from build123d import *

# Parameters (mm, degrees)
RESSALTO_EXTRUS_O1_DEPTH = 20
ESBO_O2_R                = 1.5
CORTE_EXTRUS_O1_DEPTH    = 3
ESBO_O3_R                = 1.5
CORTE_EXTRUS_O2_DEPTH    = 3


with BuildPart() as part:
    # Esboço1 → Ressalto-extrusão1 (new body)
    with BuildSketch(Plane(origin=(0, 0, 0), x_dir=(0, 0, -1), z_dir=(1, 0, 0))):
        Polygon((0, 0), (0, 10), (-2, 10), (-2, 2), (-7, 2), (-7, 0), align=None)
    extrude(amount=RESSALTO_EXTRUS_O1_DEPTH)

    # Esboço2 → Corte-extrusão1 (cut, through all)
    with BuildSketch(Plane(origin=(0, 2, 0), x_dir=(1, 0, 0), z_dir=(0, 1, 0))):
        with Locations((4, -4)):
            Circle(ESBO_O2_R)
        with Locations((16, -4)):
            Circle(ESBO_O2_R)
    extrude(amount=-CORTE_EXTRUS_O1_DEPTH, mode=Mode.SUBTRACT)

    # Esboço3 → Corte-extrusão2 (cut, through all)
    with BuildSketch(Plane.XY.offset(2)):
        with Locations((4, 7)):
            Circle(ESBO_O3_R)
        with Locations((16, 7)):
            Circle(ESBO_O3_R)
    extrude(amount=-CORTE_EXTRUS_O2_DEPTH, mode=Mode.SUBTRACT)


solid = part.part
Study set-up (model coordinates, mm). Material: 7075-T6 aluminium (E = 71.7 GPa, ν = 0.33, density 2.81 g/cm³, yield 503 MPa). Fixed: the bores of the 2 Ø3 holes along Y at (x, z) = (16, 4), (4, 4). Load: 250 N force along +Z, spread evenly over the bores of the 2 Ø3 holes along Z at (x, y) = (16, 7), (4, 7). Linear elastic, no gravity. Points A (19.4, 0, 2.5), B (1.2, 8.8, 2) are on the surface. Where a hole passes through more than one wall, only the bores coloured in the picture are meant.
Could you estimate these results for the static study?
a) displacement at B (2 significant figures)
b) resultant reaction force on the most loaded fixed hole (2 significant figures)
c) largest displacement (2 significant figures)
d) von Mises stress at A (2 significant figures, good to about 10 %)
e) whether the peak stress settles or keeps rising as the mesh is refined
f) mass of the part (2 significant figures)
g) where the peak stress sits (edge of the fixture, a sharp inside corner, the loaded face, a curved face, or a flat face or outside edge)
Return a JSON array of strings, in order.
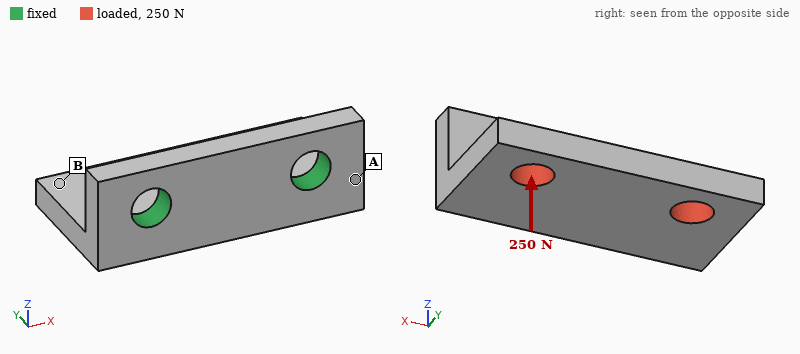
["48 µm", "130 N", "59 µm", "68 MPa", "keeps rising", "1.5 g", "edge of the fixture"]
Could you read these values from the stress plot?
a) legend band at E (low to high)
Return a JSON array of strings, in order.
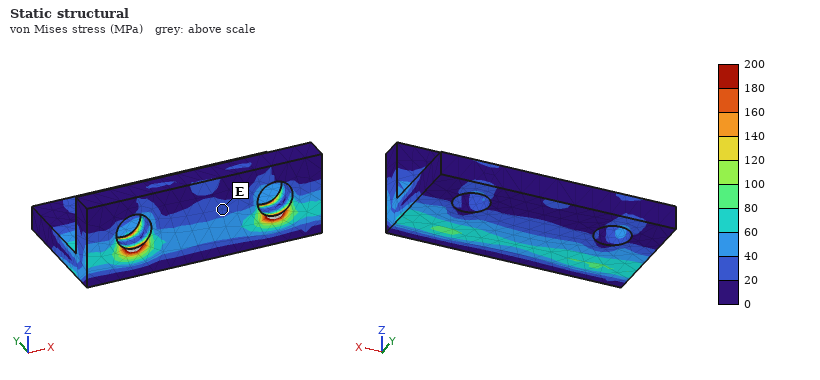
["20 to 40 MPa"]
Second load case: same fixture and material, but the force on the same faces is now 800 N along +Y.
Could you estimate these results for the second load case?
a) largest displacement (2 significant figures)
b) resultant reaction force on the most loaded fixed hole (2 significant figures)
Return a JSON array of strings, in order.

["27 µm", "400 N"]
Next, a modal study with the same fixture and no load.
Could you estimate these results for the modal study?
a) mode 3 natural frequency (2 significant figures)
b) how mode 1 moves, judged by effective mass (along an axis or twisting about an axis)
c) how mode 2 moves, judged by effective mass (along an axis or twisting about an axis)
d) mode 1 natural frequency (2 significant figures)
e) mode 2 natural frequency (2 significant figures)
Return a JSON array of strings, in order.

["42 kHz", "along Z", "twisting about Y", "16 kHz", "24 kHz"]
